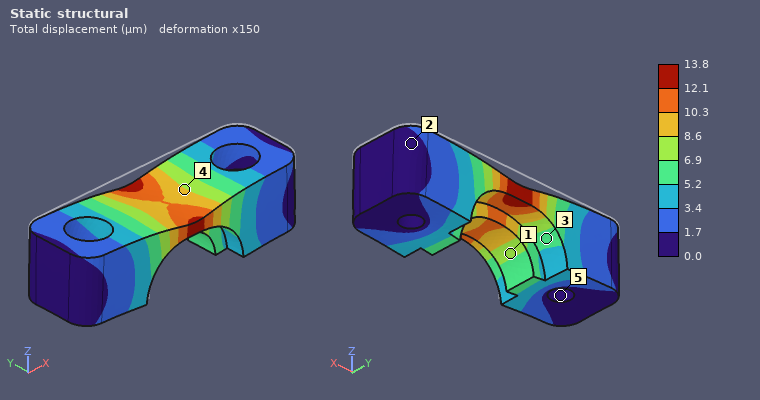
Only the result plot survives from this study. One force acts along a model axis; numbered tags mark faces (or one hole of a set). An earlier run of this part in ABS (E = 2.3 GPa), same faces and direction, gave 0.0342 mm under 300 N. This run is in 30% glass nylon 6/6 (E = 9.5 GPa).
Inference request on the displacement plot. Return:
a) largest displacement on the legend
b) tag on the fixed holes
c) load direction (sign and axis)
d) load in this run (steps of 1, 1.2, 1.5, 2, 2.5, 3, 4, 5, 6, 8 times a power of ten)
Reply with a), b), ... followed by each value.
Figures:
a) 13.8 µm
b) 5
c) -Z
d) 500 N
